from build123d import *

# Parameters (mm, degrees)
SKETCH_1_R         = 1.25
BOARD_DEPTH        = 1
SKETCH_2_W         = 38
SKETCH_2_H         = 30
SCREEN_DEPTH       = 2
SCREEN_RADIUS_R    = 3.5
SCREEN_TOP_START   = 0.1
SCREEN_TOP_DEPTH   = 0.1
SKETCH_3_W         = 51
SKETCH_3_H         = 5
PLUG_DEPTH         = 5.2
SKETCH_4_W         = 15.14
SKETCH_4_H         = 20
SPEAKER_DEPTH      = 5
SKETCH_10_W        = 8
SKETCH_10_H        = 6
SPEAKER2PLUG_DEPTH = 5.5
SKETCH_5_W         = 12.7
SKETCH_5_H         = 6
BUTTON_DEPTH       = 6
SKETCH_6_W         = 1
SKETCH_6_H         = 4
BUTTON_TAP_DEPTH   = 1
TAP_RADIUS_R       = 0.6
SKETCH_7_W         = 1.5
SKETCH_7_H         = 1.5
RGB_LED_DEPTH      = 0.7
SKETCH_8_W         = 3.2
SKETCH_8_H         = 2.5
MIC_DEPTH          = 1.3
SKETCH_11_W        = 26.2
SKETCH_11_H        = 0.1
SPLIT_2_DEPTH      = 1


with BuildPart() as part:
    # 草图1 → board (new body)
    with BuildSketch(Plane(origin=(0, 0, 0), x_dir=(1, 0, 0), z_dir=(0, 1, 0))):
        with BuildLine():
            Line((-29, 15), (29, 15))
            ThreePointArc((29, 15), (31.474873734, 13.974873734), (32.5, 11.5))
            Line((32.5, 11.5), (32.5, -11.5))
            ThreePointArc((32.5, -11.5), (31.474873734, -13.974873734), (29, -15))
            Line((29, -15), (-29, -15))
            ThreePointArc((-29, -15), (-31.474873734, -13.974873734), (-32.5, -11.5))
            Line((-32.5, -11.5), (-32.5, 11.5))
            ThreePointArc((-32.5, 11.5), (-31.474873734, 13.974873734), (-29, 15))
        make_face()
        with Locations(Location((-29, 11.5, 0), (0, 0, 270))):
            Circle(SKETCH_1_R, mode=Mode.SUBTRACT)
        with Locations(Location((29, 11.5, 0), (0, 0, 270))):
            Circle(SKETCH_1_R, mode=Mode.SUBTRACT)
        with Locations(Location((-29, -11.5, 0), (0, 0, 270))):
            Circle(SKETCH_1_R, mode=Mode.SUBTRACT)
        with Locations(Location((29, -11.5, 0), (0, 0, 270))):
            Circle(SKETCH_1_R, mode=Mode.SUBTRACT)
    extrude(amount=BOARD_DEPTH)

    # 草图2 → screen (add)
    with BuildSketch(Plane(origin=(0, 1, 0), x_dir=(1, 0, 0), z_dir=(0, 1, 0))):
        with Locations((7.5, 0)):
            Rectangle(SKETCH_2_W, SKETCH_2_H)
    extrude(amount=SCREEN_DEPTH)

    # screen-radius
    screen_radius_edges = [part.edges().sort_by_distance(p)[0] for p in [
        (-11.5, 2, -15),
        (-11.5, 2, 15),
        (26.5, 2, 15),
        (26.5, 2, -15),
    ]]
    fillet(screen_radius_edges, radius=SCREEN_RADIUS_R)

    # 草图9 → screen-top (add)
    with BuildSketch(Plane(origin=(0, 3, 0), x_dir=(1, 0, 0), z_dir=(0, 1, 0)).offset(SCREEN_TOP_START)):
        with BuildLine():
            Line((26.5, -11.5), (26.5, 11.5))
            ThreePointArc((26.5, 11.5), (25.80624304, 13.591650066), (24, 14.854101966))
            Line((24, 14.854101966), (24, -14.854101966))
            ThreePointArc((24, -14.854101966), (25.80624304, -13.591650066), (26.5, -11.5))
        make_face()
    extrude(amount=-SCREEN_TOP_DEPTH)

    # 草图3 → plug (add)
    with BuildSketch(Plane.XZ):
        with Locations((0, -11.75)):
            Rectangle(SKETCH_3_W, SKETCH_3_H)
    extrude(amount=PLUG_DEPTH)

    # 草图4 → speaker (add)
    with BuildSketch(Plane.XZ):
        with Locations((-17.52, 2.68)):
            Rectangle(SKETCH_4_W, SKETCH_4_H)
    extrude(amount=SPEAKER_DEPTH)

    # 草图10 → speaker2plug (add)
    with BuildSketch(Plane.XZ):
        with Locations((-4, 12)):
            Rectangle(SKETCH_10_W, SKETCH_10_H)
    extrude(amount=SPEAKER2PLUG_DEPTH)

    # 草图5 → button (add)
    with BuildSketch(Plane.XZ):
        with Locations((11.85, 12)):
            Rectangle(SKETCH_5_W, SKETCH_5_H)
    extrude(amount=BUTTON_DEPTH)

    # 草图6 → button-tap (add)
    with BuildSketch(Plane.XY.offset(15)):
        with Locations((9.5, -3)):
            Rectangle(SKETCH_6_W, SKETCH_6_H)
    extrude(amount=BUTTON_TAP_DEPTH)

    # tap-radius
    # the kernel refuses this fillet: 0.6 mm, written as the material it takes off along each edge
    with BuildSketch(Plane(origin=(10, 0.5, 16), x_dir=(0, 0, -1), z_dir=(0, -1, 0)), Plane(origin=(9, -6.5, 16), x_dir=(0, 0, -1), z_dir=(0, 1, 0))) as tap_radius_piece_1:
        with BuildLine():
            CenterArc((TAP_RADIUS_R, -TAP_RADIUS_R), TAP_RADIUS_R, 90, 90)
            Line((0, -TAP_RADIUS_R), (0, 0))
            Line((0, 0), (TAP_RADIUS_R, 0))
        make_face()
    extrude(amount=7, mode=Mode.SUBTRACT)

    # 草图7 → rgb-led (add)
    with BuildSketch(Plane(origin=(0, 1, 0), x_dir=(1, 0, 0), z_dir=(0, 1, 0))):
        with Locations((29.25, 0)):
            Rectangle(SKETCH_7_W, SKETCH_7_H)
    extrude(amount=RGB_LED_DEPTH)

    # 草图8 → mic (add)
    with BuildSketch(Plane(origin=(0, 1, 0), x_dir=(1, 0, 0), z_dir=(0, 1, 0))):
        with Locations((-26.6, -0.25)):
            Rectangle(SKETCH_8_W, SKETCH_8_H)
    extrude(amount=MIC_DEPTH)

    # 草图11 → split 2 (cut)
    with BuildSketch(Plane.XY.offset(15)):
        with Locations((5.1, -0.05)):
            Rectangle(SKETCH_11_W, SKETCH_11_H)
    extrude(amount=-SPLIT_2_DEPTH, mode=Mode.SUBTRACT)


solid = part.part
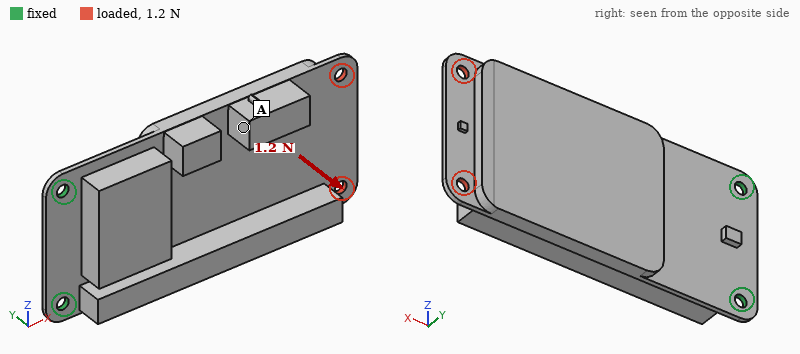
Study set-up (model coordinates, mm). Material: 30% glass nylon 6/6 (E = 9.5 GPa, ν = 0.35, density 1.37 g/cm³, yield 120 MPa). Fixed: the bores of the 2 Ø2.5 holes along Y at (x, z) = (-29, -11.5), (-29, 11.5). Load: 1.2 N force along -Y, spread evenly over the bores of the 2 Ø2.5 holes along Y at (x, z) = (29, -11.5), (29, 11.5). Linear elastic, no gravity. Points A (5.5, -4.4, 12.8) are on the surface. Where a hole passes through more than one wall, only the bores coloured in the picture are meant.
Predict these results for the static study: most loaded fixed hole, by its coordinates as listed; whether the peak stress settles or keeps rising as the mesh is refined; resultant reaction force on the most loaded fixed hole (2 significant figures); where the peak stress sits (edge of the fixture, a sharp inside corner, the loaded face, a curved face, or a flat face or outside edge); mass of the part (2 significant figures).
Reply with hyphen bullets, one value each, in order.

- (-29, -11.5)
- keeps rising
- 1.0 N
- edge of the fixture
- 11 g
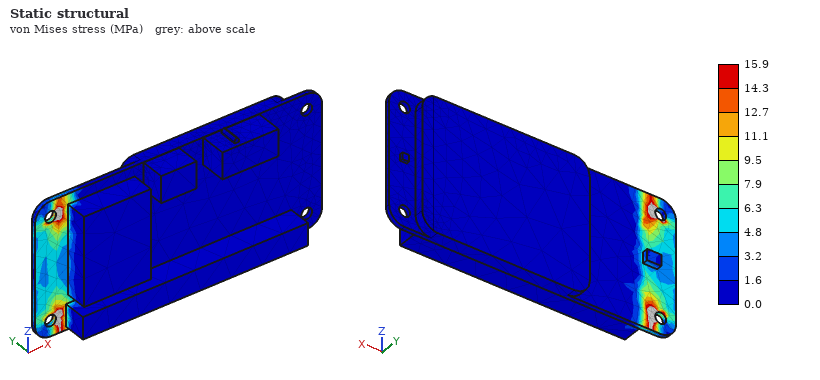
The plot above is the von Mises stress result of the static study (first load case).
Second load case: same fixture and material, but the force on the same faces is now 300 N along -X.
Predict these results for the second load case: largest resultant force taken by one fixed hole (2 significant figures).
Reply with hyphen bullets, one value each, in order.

- 150 N
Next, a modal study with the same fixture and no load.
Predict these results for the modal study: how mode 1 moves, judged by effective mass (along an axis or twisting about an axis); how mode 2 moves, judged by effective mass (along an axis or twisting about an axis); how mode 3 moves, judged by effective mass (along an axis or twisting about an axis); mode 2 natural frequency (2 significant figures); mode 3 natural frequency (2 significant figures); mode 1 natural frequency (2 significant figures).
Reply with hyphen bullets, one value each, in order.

- along Y
- twisting about X
- along Z
- 1400 Hz
- 1900 Hz
- 120 Hz
